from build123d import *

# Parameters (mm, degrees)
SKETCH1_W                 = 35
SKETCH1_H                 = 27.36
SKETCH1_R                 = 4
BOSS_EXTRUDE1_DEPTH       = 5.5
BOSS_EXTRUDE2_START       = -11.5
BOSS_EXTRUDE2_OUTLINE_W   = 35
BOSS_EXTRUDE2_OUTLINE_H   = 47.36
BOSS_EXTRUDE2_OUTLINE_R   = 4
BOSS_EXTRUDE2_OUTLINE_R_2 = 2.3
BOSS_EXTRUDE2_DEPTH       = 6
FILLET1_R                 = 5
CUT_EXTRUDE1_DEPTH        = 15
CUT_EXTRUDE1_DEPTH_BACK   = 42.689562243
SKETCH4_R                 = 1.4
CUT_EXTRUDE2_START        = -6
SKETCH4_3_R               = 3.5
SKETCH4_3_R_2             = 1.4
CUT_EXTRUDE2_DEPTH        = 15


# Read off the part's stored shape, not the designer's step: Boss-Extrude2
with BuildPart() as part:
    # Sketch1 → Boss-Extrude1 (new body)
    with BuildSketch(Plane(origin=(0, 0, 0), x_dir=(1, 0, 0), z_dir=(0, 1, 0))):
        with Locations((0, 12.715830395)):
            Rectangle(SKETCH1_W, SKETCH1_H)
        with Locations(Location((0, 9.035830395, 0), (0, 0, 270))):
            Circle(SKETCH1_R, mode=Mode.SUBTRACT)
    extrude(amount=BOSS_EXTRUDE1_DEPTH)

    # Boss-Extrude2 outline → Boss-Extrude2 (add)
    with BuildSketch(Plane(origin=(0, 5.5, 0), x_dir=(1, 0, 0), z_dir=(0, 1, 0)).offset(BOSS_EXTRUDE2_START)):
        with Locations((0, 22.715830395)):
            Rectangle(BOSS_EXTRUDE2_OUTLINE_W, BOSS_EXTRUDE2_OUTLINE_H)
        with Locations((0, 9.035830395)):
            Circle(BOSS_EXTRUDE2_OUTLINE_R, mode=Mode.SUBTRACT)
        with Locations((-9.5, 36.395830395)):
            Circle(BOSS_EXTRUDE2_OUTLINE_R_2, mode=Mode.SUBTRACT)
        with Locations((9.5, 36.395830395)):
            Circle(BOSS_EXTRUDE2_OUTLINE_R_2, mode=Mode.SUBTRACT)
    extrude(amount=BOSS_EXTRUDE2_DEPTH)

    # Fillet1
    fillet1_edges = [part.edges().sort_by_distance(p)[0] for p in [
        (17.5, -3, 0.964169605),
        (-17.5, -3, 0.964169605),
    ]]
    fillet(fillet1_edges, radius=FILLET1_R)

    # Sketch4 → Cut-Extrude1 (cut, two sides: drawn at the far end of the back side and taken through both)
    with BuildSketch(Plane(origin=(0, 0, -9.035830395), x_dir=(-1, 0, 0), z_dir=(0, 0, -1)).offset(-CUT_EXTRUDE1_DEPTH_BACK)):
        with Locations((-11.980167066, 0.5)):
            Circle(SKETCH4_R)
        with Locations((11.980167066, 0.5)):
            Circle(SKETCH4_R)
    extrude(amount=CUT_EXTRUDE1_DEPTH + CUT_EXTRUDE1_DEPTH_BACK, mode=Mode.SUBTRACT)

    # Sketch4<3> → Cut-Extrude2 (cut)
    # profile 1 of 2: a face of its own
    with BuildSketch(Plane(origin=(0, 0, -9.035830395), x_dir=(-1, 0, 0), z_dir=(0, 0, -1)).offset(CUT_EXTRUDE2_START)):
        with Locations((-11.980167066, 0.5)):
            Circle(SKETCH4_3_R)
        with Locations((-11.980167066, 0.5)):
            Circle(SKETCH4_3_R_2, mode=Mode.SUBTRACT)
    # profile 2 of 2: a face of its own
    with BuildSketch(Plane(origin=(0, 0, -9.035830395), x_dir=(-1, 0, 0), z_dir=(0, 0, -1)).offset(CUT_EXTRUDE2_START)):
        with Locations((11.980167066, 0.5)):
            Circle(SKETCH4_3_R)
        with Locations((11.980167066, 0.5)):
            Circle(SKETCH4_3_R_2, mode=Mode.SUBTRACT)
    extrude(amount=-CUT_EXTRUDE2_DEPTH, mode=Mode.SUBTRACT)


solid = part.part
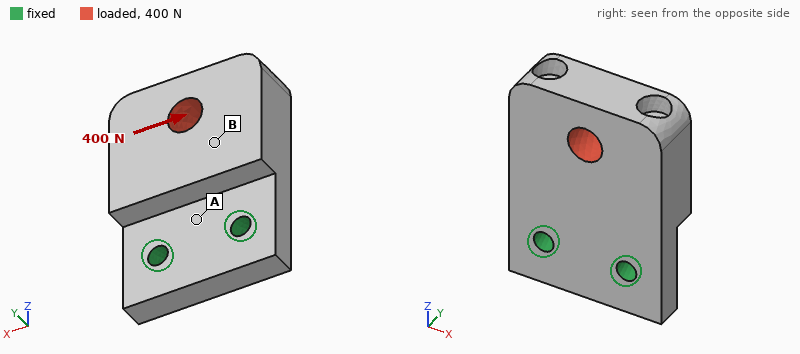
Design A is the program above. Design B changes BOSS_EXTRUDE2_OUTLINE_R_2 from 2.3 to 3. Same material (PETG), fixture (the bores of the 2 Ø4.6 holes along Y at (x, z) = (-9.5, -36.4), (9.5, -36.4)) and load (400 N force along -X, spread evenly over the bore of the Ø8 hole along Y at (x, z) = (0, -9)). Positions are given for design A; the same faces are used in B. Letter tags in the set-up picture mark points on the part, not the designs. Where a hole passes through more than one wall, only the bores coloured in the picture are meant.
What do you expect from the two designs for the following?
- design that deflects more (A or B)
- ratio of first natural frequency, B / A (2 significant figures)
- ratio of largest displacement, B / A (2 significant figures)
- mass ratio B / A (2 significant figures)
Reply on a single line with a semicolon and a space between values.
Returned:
A; 1.1; 0.89; 0.99
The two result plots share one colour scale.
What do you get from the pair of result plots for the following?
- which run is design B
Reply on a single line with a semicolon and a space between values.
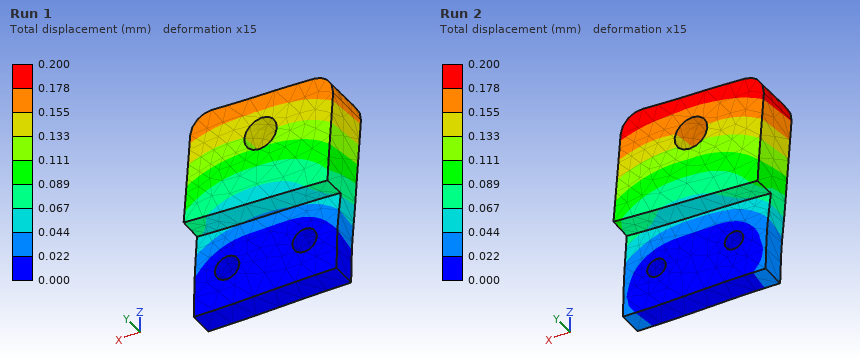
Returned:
Run 1
